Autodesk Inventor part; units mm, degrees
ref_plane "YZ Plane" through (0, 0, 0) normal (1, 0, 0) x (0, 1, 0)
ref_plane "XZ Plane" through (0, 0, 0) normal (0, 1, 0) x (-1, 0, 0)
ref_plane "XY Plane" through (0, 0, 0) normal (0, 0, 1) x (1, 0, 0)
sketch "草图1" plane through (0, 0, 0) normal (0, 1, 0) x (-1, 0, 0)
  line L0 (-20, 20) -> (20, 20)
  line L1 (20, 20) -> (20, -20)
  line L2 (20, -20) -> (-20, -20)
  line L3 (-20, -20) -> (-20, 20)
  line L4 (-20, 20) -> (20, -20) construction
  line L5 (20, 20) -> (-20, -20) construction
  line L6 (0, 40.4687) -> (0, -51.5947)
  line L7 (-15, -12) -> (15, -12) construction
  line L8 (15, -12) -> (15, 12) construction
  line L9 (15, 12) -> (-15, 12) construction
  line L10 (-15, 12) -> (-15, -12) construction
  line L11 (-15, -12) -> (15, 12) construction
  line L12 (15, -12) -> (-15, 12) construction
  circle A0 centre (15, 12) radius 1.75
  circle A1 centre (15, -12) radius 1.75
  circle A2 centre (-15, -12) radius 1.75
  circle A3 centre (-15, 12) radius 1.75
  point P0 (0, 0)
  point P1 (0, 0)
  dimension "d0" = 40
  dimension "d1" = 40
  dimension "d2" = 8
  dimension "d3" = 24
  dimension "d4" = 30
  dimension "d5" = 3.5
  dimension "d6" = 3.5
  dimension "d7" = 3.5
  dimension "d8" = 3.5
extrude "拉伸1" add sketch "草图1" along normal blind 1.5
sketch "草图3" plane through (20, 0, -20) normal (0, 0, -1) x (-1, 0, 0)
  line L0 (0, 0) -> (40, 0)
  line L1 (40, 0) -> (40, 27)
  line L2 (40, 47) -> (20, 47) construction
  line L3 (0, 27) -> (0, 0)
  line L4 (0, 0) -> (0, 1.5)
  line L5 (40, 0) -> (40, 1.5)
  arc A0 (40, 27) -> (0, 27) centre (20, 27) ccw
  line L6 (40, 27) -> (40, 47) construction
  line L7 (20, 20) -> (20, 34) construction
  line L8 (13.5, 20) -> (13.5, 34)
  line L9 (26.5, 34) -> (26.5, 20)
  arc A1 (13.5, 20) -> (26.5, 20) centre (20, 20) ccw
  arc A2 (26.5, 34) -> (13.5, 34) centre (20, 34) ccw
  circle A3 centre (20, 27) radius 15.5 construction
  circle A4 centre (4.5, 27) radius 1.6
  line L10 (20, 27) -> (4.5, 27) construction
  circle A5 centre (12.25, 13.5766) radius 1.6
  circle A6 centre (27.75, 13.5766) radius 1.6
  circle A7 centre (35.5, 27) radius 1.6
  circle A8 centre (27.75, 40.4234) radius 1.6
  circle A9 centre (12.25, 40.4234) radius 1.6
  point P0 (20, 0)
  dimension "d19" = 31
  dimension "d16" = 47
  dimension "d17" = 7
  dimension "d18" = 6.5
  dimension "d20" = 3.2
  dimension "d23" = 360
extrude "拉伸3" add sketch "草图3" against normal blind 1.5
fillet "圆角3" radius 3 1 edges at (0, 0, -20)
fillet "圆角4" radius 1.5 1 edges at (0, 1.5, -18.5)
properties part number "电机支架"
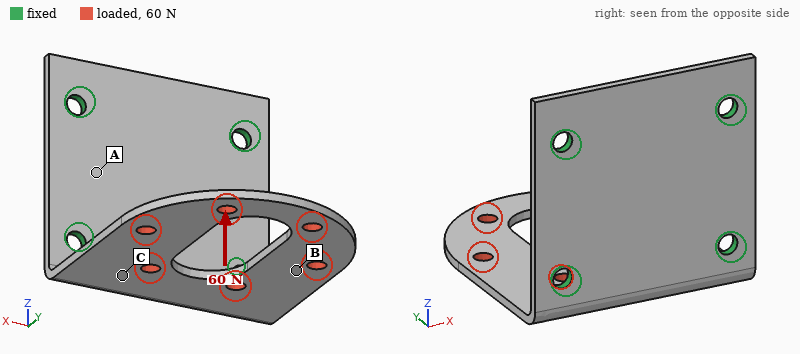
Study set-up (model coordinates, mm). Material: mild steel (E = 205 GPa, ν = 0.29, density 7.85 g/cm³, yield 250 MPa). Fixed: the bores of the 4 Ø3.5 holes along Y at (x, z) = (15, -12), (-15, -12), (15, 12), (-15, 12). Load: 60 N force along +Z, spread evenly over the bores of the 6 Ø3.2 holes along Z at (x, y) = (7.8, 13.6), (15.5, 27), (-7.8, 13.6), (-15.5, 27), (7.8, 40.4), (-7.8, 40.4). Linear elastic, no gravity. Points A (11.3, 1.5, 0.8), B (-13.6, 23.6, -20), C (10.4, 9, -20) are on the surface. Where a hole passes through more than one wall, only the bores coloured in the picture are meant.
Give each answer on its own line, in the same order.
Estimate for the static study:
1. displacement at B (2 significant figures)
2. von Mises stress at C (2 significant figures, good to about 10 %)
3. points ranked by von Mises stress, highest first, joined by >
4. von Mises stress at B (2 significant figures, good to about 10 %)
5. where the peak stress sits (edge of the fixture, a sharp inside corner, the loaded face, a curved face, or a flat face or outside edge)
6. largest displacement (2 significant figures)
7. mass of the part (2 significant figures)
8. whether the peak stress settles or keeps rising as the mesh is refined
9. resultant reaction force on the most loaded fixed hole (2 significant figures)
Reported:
0.23 mm
67 MPa
C > B > A
41 MPa
edge of the fixture
0.62 mm
33 g
keeps rising
20 N
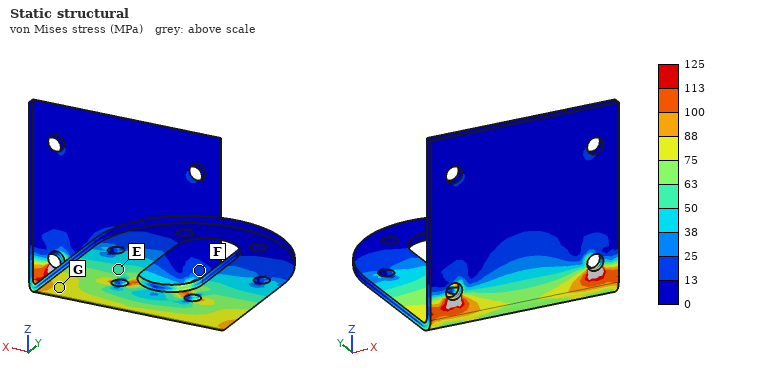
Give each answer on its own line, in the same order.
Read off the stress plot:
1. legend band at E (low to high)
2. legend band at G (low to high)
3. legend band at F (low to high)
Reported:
50 to 63 MPa
75 to 88 MPa
13 to 25 MPa
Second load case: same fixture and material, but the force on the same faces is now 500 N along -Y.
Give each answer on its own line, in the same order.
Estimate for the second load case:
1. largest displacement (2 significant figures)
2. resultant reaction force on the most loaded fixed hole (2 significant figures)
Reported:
0.24 mm
260 N
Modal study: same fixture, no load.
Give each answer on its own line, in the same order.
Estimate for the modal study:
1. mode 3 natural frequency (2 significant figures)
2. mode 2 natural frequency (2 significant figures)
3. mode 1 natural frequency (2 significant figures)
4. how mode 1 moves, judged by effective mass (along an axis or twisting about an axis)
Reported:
3100 Hz
1600 Hz
610 Hz
along Z
